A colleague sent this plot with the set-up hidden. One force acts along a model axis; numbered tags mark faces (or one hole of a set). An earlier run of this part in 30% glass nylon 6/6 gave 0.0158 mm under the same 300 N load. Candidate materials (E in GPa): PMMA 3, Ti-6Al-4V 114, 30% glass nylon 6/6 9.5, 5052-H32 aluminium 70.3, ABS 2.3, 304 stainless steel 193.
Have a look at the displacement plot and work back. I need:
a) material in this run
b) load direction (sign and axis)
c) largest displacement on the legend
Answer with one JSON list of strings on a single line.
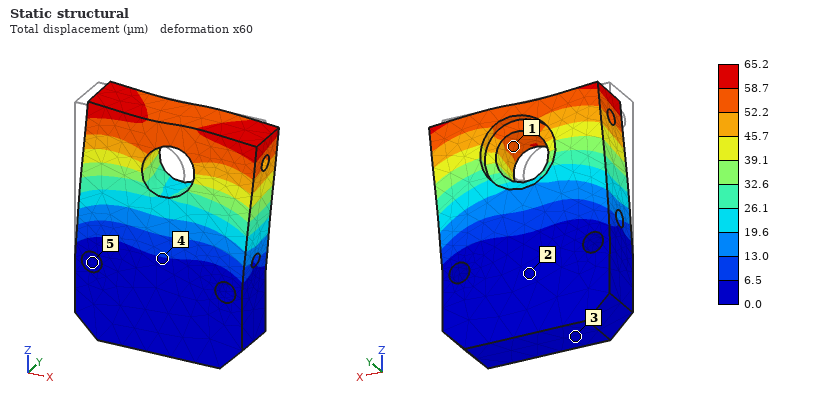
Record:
["ABS", "+X", "65.2 µm"]
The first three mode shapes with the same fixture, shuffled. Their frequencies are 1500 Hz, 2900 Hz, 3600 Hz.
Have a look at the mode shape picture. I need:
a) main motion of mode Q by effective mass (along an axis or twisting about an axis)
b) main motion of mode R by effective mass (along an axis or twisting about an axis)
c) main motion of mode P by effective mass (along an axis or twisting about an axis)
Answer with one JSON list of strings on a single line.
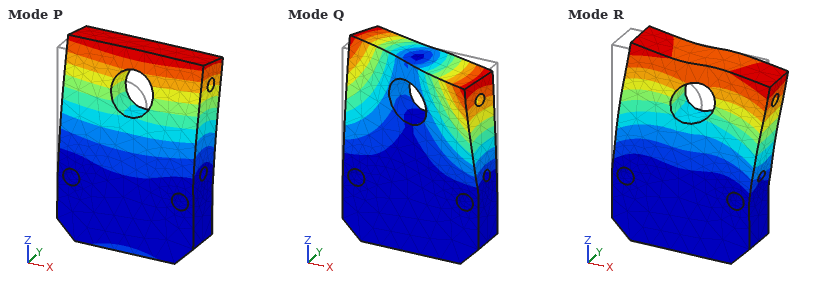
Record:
["twisting about Z", "along X", "along Y"]
